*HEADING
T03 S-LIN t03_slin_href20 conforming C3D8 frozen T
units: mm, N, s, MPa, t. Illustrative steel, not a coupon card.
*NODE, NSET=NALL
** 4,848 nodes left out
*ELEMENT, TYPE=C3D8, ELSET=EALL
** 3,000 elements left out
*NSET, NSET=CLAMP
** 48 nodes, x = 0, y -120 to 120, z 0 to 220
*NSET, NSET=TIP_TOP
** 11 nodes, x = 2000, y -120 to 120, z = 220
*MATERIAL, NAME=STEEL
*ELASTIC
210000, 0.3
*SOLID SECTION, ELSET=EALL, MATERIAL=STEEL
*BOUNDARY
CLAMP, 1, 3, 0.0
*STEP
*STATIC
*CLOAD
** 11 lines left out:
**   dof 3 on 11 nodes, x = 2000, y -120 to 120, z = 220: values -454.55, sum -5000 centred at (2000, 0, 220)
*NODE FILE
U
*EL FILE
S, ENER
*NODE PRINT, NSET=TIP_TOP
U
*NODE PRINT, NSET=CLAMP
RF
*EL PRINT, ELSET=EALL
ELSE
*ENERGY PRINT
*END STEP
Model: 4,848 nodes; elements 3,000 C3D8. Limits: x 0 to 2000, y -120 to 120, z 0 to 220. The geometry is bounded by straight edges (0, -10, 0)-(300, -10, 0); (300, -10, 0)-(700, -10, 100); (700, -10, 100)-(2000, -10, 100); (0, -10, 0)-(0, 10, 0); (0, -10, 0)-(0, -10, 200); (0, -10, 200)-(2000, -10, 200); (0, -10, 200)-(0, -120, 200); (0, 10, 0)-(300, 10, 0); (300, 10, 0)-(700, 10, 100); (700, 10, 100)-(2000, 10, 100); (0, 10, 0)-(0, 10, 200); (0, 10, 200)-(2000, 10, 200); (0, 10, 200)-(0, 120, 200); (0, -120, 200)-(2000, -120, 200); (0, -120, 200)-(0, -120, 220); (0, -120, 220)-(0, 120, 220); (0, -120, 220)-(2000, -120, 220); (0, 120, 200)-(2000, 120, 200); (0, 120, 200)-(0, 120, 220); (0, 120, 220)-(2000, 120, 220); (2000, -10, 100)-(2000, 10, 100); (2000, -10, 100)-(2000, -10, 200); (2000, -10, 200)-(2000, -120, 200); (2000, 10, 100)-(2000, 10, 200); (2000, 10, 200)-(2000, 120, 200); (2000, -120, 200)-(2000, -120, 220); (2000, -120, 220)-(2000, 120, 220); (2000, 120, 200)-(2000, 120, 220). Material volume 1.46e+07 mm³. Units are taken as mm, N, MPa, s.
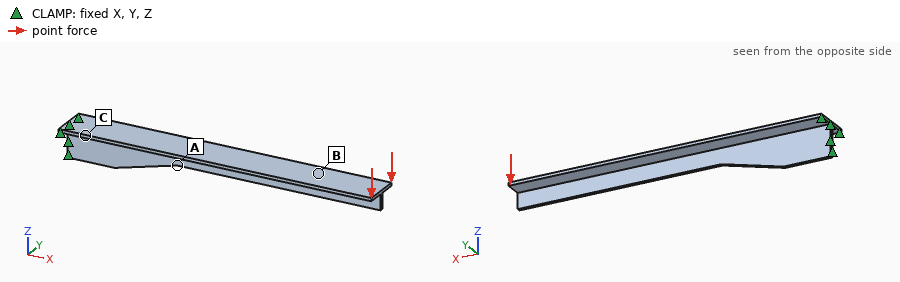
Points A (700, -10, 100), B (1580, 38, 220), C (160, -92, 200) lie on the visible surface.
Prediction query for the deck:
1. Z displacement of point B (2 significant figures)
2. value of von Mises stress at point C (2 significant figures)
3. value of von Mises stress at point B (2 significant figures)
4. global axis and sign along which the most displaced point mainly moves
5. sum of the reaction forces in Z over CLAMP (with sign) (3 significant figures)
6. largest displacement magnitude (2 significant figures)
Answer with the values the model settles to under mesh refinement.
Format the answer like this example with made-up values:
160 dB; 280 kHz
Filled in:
-2.8 mm; 9.2 MPa; 8.6 MPa; -Z; 5000 N; 4.5 mm
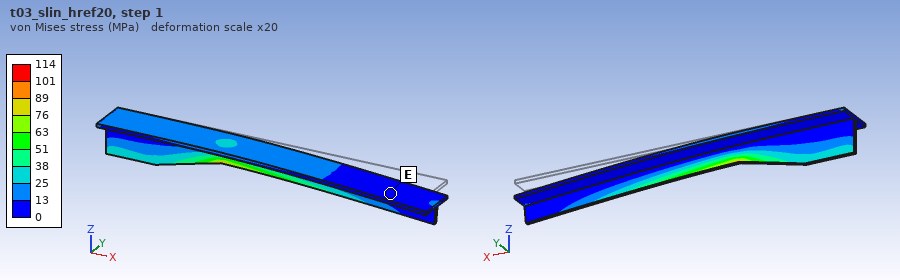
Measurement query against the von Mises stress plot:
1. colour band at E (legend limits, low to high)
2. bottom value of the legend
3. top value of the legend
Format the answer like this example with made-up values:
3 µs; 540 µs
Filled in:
0 to 13 MPa; 0 MPa; 114 MPa
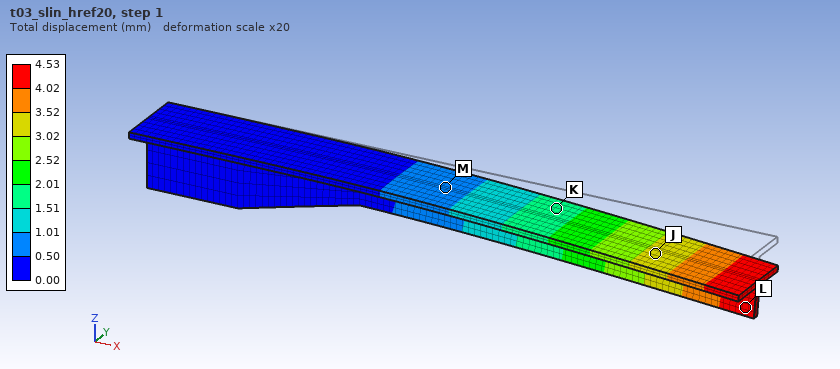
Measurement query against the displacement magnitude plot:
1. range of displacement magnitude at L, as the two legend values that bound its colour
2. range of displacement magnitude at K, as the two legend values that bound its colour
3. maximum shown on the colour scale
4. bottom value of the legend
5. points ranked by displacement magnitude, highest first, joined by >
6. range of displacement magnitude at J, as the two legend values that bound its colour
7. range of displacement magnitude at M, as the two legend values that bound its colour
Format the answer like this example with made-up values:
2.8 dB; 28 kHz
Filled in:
4.02 to 4.53 mm; 1.51 to 2.01 mm; 4.53 mm; 0.00 mm; L > J > K > M; 3.02 to 3.52 mm; 0.50 to 1.01 mm
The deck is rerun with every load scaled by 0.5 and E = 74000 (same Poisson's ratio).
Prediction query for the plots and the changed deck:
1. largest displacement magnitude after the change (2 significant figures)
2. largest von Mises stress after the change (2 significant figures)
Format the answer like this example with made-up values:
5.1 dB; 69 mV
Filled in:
6.4 mm; 57 MPa
